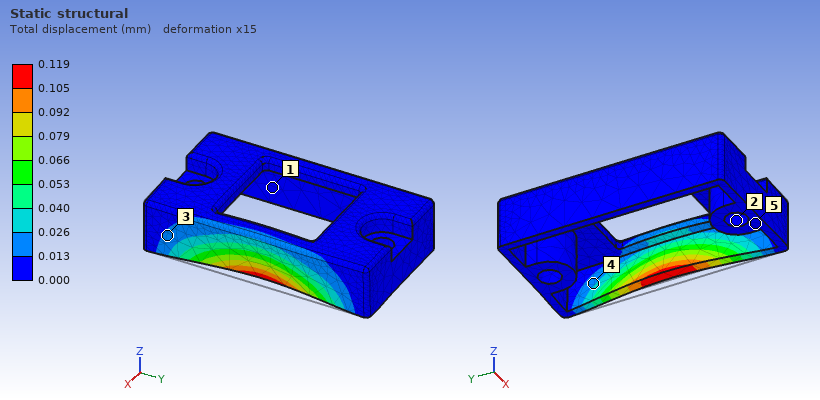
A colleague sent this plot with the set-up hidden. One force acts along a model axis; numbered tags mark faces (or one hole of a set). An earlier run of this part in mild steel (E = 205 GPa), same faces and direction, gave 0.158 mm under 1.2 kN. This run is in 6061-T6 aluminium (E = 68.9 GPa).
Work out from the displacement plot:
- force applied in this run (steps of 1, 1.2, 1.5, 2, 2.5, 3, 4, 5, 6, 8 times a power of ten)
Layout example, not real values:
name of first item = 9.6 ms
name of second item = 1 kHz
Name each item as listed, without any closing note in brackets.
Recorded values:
force applied in this run = 300 N
